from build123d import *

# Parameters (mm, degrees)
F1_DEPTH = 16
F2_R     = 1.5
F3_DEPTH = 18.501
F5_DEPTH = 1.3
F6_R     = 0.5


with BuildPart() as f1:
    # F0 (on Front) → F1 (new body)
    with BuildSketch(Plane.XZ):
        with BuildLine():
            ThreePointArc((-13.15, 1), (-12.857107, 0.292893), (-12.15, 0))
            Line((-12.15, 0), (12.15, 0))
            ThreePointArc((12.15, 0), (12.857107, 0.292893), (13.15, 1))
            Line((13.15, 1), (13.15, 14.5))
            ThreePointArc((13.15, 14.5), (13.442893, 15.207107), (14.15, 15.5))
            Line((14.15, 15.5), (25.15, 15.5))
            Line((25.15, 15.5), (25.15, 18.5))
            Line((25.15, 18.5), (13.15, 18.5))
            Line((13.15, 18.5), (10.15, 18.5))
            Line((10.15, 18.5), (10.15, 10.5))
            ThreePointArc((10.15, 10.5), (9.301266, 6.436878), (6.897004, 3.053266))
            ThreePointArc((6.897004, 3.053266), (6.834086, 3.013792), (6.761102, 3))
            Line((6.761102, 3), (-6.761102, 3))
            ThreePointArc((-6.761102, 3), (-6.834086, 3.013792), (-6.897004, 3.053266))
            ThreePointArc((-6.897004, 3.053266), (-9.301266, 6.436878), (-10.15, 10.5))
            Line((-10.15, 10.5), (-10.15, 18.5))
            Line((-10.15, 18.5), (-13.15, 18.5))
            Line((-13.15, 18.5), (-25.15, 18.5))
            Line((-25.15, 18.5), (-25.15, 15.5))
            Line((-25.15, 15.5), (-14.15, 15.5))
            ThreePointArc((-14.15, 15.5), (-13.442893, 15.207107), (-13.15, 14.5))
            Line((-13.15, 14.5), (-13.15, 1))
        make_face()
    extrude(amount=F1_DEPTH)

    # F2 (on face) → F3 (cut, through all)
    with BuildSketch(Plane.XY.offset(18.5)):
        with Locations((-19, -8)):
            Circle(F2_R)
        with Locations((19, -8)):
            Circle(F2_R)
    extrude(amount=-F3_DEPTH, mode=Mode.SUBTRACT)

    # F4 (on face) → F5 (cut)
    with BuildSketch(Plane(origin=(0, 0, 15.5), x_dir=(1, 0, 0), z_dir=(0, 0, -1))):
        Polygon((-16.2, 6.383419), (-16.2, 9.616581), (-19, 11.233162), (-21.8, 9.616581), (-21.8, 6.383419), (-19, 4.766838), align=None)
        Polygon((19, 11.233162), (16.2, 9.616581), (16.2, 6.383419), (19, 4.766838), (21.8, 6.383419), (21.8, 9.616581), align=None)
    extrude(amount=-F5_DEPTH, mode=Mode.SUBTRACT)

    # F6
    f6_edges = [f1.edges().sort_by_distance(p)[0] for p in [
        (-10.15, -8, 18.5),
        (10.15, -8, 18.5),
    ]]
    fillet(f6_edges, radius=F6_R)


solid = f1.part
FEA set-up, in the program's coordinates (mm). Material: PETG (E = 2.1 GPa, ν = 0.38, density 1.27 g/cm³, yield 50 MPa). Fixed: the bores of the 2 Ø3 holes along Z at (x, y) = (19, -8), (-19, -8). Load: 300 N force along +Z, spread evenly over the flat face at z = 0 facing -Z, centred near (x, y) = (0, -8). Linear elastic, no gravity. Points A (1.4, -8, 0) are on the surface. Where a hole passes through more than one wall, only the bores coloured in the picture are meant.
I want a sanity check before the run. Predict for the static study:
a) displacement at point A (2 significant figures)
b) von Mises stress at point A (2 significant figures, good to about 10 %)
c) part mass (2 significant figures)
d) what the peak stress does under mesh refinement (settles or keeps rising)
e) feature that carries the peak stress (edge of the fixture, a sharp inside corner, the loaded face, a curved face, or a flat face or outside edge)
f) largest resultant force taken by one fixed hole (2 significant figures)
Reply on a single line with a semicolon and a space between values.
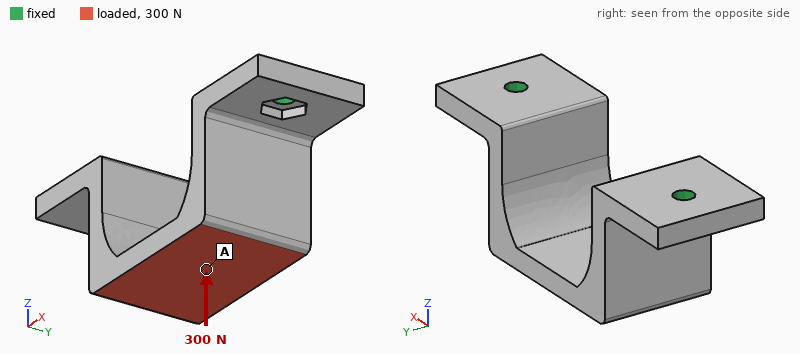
0.25 mm; 6.4 MPa; 5.1 g; keeps rising; edge of the fixture; 170 N
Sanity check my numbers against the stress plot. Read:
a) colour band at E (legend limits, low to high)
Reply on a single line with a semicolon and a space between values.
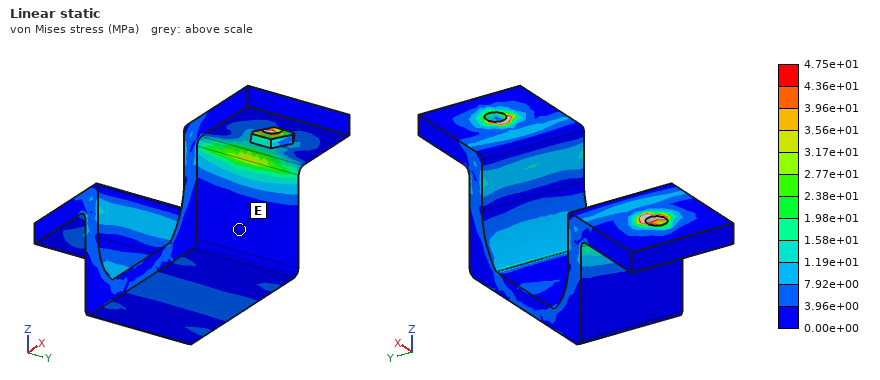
0.00e+00 to 3.96e+00 MPa
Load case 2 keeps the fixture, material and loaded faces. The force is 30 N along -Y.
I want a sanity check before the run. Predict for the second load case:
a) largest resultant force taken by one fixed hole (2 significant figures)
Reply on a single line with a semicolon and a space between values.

15 N
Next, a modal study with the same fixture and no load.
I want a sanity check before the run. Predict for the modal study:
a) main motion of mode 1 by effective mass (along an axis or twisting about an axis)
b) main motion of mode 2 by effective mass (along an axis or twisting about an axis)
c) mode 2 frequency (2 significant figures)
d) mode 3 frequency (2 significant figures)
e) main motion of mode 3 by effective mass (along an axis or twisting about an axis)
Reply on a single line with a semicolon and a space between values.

along Y; along X; 2000 Hz; 2300 Hz; twisting about Z
